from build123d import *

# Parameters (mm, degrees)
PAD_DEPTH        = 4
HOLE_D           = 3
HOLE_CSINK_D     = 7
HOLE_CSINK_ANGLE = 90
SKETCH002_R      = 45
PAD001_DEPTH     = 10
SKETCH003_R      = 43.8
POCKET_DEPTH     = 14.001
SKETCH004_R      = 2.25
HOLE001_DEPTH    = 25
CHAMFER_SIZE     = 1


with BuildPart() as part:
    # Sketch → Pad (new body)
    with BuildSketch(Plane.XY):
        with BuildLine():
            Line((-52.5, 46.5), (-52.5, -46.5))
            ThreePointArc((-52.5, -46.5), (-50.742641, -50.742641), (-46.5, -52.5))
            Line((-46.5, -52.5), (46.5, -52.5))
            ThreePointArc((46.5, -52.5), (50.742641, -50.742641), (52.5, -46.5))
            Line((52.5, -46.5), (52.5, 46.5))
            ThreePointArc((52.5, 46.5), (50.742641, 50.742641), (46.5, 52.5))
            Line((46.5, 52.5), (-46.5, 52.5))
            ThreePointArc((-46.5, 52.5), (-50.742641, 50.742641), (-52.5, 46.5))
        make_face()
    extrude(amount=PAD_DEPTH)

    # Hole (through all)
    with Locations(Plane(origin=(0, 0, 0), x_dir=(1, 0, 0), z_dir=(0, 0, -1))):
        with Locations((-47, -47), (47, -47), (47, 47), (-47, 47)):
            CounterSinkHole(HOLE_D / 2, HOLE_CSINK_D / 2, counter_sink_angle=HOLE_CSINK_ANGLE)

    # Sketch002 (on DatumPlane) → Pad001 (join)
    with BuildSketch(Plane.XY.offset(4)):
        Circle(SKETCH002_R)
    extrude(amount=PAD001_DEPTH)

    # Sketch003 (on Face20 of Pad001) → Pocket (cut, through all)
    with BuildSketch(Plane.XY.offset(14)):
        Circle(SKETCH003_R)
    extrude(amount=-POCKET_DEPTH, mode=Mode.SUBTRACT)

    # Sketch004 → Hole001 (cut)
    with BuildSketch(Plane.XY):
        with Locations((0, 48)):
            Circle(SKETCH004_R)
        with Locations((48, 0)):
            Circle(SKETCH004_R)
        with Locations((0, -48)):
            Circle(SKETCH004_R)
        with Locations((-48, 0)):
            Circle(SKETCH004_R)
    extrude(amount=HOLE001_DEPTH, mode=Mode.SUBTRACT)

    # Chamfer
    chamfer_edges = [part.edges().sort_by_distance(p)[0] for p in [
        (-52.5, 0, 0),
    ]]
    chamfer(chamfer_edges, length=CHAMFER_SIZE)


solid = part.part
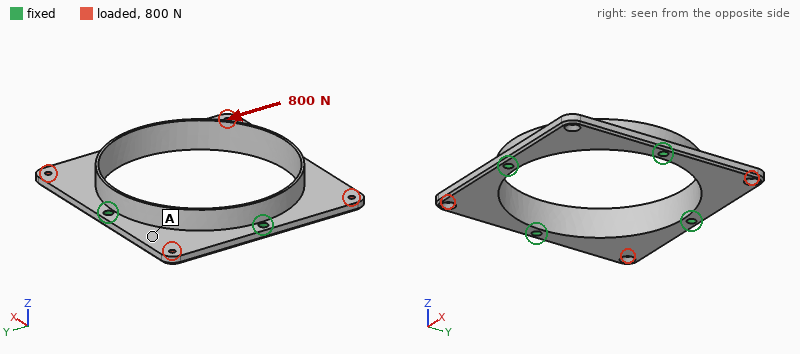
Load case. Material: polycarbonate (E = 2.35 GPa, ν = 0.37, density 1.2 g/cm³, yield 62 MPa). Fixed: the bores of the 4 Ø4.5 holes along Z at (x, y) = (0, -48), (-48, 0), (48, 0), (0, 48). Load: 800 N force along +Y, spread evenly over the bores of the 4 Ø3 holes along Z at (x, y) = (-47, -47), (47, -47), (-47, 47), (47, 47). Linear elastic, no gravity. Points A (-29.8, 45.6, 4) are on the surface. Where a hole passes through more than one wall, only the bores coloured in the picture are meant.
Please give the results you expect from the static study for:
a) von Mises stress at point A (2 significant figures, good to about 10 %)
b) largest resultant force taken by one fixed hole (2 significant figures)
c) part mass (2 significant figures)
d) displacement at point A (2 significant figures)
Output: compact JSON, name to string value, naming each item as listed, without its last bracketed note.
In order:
{"von Mises stress at point A": "1.5 MPa", "largest resultant force taken by one fixed hole": "400 N", "part mass": "27 g", "displacement at point A": "0.11 mm"}
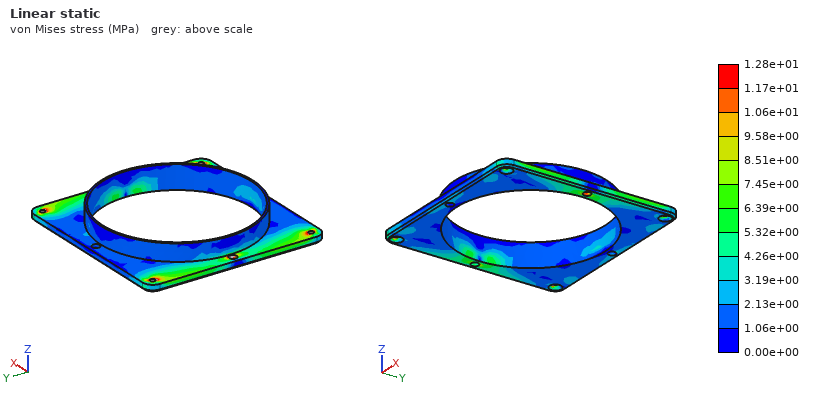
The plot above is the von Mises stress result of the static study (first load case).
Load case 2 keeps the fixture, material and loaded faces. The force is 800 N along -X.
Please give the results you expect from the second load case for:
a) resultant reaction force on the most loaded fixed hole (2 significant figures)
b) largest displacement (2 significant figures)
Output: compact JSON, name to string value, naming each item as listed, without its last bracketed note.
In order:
{"resultant reaction force on the most loaded fixed hole": "400 N", "largest displacement": "0.33 mm"}
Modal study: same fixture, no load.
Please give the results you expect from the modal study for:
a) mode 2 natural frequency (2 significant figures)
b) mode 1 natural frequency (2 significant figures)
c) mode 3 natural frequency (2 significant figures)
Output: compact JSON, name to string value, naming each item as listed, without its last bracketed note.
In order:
{"mode 2 natural frequency": "640 Hz", "mode 1 natural frequency": "590 Hz", "mode 3 natural frequency": "640 Hz"}
